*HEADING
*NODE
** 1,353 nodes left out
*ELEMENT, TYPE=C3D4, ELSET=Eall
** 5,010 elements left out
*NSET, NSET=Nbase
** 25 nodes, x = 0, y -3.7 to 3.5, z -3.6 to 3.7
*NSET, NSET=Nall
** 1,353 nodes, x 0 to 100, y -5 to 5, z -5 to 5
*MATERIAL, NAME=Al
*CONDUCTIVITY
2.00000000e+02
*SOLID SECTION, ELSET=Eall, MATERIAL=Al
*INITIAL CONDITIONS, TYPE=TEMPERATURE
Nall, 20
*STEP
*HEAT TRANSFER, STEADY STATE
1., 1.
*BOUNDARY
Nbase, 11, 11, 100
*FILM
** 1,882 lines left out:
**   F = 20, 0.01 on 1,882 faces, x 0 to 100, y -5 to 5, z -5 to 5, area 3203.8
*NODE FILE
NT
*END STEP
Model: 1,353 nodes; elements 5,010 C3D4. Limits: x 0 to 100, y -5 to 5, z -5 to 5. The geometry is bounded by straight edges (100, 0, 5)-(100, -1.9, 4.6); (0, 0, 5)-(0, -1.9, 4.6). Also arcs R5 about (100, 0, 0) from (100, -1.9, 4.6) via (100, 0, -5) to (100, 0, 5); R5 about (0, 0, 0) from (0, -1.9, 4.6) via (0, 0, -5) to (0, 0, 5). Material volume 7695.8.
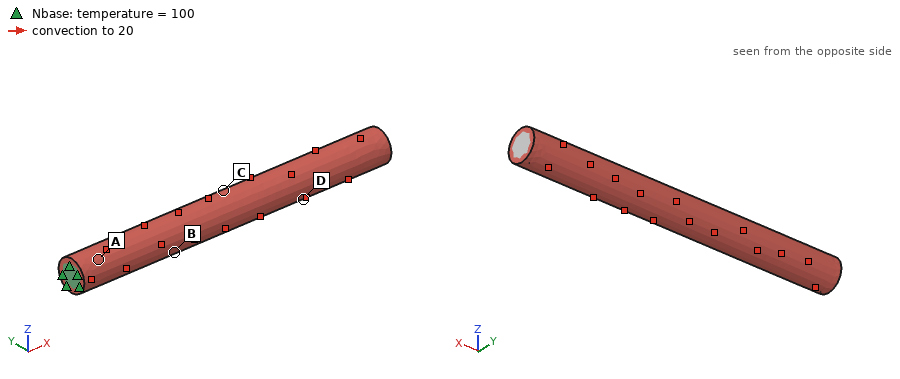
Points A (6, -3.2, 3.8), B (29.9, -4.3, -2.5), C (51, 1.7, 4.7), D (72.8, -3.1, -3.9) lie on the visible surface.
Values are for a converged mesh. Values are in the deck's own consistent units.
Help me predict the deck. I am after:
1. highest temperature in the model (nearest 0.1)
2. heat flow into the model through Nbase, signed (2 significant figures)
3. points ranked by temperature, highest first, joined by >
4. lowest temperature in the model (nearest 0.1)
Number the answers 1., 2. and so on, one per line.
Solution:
1. 100.0
2. 2400
3. A > B > C > D
4. 92.3
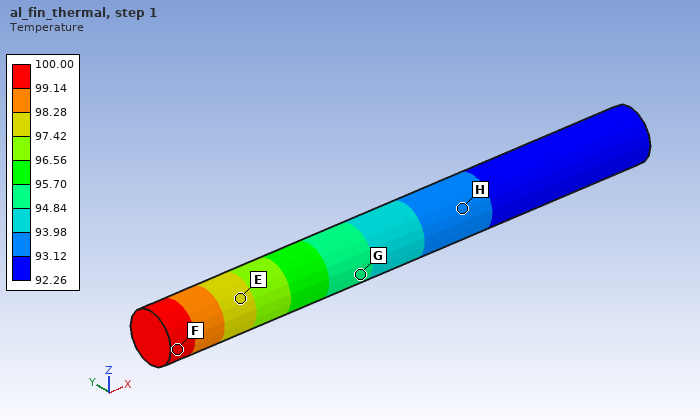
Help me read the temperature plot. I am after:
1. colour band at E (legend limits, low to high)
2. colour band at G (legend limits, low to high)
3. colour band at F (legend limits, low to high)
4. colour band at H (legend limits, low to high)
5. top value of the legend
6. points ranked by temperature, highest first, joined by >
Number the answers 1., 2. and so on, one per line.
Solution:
1. 97.42 to 98.28
2. 94.84 to 95.70
3. 99.14 to 100.00
4. 93.12 to 93.98
5. 100.00
6. F > E > G > H
